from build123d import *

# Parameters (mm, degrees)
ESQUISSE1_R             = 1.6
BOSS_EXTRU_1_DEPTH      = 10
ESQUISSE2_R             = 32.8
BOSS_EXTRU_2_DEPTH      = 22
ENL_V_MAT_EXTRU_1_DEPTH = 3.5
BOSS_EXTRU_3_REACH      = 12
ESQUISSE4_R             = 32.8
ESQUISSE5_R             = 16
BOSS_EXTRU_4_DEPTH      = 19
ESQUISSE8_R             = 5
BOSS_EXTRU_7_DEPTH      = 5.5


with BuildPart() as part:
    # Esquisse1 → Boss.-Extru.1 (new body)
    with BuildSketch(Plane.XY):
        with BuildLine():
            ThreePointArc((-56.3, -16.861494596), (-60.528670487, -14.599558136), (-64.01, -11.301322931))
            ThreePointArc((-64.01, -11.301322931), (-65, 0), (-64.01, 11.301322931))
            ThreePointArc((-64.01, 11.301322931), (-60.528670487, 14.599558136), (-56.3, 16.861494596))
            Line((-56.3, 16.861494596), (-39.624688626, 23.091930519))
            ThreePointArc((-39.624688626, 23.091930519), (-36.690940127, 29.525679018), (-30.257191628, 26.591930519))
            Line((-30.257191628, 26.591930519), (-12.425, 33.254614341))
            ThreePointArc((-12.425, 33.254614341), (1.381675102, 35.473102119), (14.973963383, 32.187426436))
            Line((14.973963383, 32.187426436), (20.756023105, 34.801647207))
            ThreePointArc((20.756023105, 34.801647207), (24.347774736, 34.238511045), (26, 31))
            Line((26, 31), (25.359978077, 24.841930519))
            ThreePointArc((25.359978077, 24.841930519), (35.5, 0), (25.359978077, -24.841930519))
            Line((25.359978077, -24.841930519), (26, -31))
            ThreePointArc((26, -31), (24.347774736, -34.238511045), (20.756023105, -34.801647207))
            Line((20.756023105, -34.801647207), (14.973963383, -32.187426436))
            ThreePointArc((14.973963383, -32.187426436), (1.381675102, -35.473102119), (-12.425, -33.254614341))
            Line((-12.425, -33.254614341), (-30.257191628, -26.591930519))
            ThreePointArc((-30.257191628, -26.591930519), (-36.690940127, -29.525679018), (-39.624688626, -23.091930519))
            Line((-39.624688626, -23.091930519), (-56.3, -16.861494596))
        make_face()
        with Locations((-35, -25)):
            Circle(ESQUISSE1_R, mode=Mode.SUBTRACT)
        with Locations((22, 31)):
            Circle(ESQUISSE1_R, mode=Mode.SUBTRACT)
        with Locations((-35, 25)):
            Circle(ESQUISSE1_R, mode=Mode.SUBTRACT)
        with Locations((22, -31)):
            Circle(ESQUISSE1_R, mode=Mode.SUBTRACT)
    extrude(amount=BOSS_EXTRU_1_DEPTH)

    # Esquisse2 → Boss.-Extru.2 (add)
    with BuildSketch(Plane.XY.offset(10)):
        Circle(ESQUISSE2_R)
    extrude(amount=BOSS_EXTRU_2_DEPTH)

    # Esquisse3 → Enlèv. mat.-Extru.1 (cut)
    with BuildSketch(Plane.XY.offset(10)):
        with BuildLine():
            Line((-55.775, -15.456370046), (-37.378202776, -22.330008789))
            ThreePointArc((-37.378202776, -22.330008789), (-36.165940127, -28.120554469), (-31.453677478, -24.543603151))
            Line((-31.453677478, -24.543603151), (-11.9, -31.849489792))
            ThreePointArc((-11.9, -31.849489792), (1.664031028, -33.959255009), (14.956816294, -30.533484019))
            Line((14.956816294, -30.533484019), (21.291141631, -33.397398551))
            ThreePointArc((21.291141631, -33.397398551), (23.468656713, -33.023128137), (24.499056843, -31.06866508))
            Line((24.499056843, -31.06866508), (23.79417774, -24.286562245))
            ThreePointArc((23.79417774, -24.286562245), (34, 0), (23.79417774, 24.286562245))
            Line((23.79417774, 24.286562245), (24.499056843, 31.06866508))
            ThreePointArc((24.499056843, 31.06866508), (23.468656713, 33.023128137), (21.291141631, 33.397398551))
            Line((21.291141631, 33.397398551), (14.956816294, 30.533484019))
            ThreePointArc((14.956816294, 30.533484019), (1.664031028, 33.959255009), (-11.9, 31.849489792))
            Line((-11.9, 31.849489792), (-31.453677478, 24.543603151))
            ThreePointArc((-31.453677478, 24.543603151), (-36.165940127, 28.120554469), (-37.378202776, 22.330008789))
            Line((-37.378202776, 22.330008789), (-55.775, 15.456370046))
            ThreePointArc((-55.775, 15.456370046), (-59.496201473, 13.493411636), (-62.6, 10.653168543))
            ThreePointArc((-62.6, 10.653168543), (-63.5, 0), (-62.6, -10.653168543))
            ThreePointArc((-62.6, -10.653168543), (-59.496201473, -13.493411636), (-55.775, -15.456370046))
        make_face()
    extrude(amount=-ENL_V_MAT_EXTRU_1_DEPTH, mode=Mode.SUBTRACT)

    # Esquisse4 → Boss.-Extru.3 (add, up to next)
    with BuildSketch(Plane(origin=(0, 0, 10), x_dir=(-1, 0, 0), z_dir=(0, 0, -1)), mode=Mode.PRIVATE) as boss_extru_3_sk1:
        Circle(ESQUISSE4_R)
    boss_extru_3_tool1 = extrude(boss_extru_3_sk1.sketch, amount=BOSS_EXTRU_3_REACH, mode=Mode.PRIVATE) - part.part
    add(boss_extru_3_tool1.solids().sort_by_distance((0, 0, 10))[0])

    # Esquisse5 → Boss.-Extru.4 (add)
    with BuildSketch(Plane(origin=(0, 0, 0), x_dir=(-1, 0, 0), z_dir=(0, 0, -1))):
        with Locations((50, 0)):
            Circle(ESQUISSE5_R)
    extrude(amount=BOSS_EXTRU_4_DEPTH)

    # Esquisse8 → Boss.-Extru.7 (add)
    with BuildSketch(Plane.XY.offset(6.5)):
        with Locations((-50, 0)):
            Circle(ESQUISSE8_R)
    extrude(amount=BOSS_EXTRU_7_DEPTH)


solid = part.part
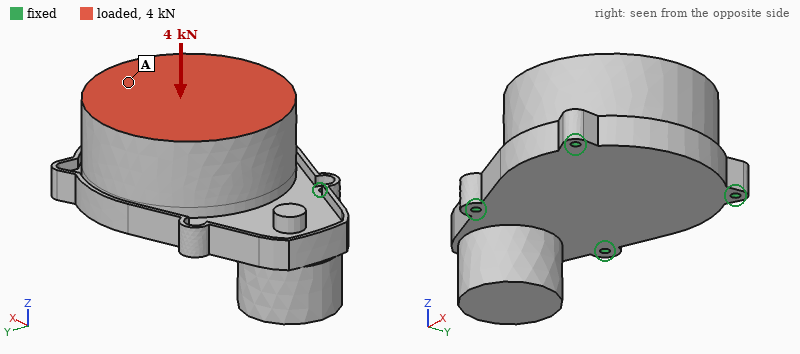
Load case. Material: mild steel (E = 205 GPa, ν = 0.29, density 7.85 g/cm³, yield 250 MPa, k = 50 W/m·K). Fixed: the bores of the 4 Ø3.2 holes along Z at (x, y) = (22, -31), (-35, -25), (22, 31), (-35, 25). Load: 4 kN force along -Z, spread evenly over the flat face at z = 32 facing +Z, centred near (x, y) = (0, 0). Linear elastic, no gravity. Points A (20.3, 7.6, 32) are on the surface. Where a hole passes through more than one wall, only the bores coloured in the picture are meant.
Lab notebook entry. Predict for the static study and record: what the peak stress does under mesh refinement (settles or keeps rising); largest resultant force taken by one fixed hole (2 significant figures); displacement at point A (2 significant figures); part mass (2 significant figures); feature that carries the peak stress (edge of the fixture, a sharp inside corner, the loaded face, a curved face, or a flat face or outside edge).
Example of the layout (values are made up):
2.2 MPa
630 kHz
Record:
keeps rising
1.3 kN
3.1 µm
1.1 kg
edge of the fixture
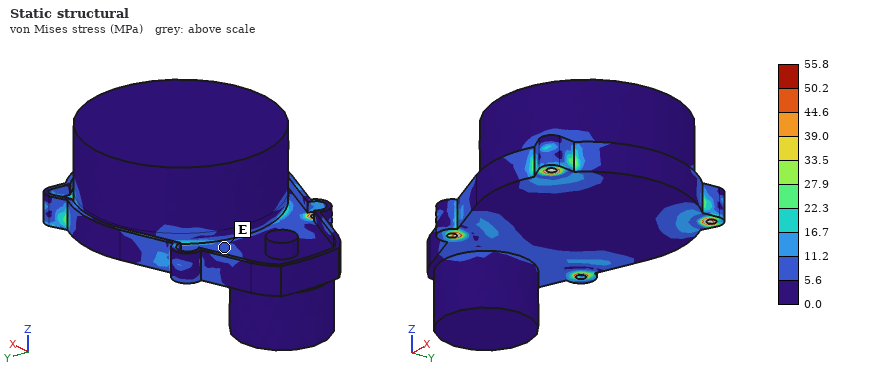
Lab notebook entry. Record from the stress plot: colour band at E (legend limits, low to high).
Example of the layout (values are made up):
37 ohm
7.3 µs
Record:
5.6 to 11.2 MPa
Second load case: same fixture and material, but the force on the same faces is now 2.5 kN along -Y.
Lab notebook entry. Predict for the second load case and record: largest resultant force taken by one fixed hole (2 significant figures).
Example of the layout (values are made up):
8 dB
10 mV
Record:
1.3 kN
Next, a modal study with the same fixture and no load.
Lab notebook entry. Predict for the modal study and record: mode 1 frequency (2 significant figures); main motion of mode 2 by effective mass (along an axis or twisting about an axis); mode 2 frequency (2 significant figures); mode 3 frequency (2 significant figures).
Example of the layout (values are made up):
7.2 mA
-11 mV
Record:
2900 Hz
along Z
5700 Hz
6500 Hz
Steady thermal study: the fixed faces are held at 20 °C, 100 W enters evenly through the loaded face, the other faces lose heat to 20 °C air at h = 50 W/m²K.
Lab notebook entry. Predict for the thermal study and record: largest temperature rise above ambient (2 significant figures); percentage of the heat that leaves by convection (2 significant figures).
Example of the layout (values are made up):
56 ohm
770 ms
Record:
57 K
31 %
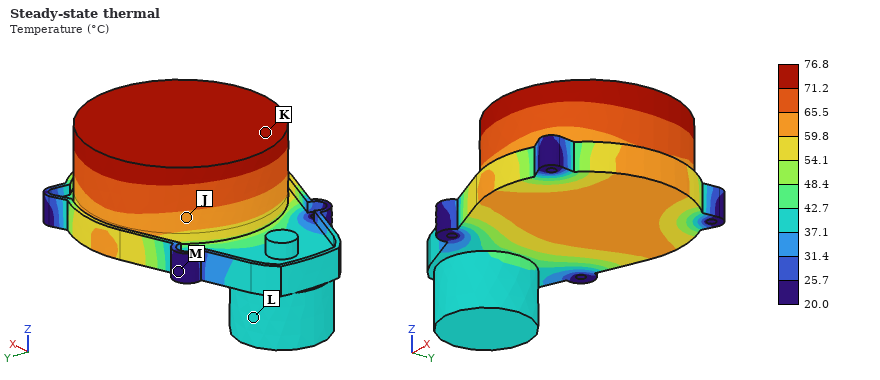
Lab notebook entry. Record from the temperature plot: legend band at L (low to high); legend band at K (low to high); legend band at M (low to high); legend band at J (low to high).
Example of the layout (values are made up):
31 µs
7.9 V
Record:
37.1 to 42.7 °C
71.2 to 76.8 °C
20.0 to 25.7 °C
59.8 to 65.5 °C
